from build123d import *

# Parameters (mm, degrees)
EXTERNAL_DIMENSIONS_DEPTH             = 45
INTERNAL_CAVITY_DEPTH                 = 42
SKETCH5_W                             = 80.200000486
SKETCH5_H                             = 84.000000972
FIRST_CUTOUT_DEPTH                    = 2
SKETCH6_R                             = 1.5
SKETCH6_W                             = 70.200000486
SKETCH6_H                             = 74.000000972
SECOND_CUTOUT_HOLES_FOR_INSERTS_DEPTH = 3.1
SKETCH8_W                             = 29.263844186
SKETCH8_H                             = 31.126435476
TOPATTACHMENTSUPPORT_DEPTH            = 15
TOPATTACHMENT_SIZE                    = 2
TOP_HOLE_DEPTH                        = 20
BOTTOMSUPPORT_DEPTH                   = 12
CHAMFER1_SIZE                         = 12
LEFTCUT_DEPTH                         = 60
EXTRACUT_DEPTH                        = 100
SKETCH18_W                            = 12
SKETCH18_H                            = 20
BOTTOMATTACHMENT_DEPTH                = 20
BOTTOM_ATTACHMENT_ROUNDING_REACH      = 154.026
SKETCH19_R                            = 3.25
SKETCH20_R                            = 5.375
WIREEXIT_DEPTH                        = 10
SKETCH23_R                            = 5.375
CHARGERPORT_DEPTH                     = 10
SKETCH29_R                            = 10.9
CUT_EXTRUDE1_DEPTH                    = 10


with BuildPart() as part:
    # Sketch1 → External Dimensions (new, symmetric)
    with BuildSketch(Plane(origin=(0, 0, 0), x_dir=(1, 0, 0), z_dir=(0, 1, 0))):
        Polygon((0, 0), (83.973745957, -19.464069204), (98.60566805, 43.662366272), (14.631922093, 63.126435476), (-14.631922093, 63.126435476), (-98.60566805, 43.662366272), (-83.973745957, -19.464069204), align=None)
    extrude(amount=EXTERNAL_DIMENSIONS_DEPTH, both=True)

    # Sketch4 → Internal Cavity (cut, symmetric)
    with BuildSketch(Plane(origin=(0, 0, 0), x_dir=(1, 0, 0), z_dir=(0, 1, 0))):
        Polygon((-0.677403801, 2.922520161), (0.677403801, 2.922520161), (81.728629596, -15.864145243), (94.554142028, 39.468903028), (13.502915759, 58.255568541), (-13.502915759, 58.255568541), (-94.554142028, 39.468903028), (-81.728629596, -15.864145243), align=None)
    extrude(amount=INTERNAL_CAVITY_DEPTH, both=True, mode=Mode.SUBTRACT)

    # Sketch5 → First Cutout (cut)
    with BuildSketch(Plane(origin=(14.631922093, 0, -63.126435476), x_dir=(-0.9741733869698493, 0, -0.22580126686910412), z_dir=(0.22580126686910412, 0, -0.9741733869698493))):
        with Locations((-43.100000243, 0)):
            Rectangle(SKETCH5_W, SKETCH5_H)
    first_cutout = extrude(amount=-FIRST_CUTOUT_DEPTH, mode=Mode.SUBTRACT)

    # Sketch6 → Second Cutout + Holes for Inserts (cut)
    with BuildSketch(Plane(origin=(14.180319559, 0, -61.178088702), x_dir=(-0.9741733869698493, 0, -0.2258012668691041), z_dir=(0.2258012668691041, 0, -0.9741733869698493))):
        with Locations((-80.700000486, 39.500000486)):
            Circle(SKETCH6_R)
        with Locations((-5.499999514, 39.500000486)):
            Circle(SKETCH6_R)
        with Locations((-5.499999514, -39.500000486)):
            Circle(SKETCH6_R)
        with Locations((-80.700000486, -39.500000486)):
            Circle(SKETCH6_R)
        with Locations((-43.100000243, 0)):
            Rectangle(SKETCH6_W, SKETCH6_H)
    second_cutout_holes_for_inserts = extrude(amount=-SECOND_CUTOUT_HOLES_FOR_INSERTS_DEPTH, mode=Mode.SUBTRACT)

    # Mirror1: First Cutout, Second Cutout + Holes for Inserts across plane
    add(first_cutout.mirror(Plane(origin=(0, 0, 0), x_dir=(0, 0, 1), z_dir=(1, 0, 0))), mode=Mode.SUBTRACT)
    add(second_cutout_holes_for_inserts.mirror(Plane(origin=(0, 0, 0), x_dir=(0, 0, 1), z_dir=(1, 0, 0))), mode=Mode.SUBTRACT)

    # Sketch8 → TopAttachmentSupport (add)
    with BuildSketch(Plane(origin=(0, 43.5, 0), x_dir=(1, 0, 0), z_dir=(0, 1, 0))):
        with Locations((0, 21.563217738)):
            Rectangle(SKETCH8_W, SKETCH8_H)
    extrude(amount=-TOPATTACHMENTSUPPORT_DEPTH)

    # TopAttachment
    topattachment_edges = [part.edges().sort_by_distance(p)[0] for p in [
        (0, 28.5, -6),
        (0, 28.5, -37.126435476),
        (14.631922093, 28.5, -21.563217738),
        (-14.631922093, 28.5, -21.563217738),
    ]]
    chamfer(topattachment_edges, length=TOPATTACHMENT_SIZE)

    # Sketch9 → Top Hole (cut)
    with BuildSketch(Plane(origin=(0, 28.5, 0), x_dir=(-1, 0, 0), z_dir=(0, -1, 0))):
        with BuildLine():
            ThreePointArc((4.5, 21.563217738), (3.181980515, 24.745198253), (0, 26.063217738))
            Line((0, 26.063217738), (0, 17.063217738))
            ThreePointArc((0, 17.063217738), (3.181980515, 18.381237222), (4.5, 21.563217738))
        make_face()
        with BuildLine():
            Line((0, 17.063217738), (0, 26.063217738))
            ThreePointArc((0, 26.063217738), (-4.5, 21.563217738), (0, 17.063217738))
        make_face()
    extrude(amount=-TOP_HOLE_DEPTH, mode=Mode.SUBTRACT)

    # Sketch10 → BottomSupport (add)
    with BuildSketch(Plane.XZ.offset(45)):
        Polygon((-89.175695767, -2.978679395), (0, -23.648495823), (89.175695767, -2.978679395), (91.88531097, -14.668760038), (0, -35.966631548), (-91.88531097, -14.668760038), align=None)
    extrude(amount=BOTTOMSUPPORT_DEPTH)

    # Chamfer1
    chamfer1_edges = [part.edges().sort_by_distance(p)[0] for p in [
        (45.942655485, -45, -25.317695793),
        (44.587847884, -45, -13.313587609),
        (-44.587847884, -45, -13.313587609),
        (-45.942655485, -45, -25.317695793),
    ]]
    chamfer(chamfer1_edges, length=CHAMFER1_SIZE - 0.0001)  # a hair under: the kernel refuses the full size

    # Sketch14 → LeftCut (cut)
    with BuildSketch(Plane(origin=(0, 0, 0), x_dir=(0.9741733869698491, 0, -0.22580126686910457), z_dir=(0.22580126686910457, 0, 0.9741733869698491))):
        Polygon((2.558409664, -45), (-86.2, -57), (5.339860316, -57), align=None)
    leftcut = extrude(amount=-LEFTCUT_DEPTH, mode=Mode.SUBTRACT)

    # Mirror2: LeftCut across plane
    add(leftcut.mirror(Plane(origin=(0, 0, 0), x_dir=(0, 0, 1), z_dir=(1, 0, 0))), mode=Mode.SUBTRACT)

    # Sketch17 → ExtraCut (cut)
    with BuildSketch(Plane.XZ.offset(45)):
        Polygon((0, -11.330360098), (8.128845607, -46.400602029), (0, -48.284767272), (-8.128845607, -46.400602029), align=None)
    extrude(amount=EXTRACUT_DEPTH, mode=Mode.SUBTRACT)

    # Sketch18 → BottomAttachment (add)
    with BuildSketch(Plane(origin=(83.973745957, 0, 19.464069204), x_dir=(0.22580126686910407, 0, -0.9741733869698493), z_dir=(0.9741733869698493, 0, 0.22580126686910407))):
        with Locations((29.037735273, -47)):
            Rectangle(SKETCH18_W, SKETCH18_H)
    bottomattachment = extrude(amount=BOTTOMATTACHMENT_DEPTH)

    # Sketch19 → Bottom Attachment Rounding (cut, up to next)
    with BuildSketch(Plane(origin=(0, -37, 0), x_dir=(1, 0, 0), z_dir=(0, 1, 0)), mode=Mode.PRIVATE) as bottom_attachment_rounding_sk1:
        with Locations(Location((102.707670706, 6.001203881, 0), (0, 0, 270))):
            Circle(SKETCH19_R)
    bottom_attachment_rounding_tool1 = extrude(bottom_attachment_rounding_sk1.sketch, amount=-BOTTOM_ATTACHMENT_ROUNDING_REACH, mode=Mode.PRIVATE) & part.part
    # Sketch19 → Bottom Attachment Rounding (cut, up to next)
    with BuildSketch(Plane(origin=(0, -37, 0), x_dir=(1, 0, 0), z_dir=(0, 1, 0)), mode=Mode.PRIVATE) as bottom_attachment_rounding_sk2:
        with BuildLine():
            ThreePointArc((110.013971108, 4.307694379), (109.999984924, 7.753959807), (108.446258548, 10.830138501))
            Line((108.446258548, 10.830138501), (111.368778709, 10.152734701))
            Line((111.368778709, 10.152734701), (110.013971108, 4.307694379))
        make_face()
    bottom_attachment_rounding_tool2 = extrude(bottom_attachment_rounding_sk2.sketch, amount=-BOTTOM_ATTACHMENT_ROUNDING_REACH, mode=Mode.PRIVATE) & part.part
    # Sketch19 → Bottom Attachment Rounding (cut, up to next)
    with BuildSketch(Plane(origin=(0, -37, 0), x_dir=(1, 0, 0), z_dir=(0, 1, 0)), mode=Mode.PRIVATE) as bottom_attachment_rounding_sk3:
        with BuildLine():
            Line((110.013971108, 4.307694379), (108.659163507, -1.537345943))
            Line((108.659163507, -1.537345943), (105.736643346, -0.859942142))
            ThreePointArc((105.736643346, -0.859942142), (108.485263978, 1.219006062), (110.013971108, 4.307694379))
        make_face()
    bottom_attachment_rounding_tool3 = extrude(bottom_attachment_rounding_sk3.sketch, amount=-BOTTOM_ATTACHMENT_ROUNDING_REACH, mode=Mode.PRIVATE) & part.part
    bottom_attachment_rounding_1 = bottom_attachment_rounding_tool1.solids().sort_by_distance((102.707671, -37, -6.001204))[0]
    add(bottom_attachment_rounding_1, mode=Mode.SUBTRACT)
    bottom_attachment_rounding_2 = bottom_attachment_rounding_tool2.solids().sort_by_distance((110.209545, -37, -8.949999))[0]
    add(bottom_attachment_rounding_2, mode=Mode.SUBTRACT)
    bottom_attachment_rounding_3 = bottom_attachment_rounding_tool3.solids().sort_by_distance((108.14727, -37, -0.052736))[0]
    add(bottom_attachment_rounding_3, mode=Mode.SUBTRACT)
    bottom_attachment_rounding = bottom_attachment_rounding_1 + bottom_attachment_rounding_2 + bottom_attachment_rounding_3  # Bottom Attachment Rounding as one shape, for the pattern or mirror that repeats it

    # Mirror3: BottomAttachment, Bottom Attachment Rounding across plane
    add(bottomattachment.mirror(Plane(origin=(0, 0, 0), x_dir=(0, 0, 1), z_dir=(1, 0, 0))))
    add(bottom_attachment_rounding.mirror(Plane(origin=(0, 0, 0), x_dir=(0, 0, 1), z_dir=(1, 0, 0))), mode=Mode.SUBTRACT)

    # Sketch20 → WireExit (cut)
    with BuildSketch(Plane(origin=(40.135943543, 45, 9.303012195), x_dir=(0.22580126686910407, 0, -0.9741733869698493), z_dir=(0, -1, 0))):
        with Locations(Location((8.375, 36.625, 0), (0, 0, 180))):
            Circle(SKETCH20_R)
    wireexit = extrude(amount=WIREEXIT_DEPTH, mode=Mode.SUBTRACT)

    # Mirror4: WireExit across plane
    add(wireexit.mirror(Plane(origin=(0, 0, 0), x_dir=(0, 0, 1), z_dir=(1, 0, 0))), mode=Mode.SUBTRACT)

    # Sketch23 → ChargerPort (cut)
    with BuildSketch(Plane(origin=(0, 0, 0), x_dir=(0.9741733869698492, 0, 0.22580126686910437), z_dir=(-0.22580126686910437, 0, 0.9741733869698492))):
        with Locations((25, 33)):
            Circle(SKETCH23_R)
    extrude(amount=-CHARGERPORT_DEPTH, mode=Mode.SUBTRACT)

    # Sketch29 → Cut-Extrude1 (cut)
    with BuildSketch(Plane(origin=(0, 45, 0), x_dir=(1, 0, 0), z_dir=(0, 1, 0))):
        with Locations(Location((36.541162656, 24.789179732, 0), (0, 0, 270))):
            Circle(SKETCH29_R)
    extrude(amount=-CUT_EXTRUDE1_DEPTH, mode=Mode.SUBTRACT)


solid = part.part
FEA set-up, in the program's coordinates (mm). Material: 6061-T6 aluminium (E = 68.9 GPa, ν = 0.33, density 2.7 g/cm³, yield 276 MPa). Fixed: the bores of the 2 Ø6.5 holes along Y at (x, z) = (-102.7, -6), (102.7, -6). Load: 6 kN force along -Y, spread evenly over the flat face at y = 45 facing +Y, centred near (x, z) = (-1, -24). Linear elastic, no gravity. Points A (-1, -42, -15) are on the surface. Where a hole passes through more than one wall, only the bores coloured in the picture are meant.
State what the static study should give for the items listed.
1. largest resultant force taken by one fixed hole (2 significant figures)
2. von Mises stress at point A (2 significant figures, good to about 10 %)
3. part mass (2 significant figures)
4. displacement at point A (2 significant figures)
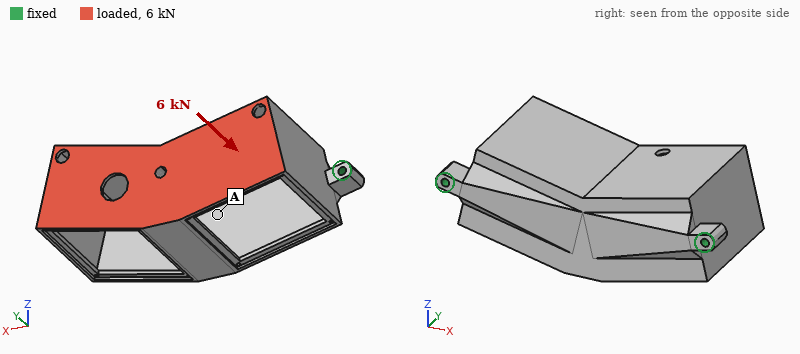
3.5 kN
16 MPa
590 g
0.12 mm
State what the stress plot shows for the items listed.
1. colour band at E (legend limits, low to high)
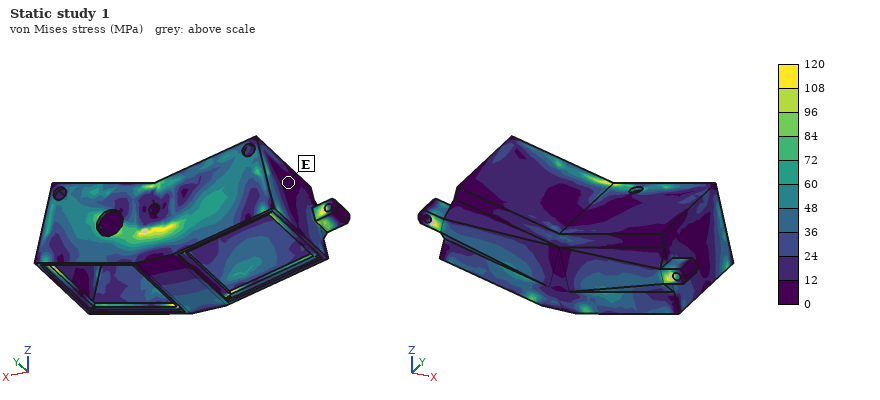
0 to 12 MPa
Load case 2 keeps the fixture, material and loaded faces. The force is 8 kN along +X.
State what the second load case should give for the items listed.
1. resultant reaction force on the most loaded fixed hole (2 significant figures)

6.0 kN
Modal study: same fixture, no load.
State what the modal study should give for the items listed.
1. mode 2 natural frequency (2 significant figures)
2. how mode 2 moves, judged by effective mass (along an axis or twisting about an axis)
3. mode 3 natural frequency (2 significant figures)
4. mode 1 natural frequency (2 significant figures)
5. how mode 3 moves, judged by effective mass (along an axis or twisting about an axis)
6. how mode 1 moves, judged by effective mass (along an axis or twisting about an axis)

970 Hz
along X
1100 Hz
560 Hz
along Y
along Z
